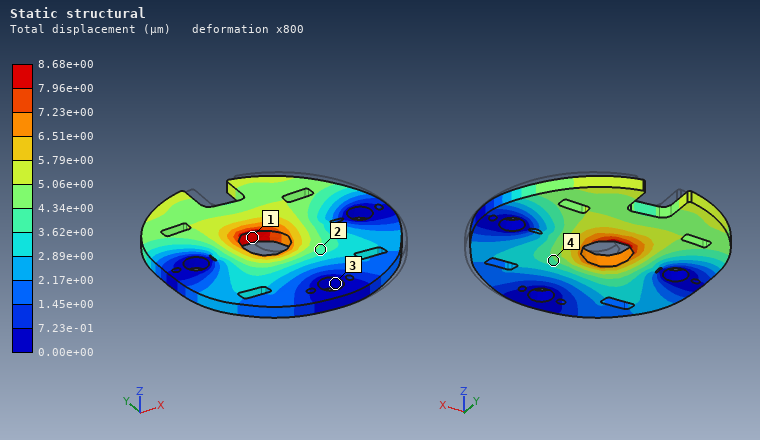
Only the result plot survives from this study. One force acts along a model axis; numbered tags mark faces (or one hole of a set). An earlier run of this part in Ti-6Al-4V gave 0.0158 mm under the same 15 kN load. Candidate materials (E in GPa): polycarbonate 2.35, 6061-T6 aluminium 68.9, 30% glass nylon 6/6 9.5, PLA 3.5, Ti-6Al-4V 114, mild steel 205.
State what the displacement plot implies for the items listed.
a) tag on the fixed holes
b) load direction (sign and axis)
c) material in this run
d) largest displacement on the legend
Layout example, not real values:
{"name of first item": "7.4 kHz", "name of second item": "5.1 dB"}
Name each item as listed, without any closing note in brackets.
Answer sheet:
{"tag on the fixed holes": "3", "load direction": "-X", "material in this run": "mild steel", "largest displacement on the legend": "8.68e+00 µm"}
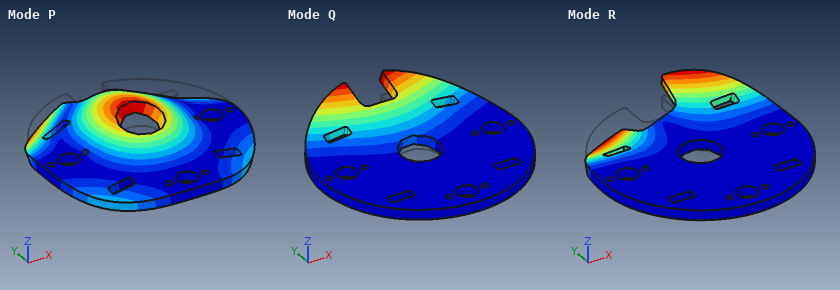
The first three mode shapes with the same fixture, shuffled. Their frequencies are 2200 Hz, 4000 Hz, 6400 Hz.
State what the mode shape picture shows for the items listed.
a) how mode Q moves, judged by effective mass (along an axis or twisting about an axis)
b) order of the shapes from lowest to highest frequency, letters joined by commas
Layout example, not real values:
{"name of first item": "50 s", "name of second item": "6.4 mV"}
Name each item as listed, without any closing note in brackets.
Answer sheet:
{"how mode Q moves, judged by effective mass": "along Z", "order of the shapes from lowest to highest frequency, letters joined by commas": "Q, R, P"}
